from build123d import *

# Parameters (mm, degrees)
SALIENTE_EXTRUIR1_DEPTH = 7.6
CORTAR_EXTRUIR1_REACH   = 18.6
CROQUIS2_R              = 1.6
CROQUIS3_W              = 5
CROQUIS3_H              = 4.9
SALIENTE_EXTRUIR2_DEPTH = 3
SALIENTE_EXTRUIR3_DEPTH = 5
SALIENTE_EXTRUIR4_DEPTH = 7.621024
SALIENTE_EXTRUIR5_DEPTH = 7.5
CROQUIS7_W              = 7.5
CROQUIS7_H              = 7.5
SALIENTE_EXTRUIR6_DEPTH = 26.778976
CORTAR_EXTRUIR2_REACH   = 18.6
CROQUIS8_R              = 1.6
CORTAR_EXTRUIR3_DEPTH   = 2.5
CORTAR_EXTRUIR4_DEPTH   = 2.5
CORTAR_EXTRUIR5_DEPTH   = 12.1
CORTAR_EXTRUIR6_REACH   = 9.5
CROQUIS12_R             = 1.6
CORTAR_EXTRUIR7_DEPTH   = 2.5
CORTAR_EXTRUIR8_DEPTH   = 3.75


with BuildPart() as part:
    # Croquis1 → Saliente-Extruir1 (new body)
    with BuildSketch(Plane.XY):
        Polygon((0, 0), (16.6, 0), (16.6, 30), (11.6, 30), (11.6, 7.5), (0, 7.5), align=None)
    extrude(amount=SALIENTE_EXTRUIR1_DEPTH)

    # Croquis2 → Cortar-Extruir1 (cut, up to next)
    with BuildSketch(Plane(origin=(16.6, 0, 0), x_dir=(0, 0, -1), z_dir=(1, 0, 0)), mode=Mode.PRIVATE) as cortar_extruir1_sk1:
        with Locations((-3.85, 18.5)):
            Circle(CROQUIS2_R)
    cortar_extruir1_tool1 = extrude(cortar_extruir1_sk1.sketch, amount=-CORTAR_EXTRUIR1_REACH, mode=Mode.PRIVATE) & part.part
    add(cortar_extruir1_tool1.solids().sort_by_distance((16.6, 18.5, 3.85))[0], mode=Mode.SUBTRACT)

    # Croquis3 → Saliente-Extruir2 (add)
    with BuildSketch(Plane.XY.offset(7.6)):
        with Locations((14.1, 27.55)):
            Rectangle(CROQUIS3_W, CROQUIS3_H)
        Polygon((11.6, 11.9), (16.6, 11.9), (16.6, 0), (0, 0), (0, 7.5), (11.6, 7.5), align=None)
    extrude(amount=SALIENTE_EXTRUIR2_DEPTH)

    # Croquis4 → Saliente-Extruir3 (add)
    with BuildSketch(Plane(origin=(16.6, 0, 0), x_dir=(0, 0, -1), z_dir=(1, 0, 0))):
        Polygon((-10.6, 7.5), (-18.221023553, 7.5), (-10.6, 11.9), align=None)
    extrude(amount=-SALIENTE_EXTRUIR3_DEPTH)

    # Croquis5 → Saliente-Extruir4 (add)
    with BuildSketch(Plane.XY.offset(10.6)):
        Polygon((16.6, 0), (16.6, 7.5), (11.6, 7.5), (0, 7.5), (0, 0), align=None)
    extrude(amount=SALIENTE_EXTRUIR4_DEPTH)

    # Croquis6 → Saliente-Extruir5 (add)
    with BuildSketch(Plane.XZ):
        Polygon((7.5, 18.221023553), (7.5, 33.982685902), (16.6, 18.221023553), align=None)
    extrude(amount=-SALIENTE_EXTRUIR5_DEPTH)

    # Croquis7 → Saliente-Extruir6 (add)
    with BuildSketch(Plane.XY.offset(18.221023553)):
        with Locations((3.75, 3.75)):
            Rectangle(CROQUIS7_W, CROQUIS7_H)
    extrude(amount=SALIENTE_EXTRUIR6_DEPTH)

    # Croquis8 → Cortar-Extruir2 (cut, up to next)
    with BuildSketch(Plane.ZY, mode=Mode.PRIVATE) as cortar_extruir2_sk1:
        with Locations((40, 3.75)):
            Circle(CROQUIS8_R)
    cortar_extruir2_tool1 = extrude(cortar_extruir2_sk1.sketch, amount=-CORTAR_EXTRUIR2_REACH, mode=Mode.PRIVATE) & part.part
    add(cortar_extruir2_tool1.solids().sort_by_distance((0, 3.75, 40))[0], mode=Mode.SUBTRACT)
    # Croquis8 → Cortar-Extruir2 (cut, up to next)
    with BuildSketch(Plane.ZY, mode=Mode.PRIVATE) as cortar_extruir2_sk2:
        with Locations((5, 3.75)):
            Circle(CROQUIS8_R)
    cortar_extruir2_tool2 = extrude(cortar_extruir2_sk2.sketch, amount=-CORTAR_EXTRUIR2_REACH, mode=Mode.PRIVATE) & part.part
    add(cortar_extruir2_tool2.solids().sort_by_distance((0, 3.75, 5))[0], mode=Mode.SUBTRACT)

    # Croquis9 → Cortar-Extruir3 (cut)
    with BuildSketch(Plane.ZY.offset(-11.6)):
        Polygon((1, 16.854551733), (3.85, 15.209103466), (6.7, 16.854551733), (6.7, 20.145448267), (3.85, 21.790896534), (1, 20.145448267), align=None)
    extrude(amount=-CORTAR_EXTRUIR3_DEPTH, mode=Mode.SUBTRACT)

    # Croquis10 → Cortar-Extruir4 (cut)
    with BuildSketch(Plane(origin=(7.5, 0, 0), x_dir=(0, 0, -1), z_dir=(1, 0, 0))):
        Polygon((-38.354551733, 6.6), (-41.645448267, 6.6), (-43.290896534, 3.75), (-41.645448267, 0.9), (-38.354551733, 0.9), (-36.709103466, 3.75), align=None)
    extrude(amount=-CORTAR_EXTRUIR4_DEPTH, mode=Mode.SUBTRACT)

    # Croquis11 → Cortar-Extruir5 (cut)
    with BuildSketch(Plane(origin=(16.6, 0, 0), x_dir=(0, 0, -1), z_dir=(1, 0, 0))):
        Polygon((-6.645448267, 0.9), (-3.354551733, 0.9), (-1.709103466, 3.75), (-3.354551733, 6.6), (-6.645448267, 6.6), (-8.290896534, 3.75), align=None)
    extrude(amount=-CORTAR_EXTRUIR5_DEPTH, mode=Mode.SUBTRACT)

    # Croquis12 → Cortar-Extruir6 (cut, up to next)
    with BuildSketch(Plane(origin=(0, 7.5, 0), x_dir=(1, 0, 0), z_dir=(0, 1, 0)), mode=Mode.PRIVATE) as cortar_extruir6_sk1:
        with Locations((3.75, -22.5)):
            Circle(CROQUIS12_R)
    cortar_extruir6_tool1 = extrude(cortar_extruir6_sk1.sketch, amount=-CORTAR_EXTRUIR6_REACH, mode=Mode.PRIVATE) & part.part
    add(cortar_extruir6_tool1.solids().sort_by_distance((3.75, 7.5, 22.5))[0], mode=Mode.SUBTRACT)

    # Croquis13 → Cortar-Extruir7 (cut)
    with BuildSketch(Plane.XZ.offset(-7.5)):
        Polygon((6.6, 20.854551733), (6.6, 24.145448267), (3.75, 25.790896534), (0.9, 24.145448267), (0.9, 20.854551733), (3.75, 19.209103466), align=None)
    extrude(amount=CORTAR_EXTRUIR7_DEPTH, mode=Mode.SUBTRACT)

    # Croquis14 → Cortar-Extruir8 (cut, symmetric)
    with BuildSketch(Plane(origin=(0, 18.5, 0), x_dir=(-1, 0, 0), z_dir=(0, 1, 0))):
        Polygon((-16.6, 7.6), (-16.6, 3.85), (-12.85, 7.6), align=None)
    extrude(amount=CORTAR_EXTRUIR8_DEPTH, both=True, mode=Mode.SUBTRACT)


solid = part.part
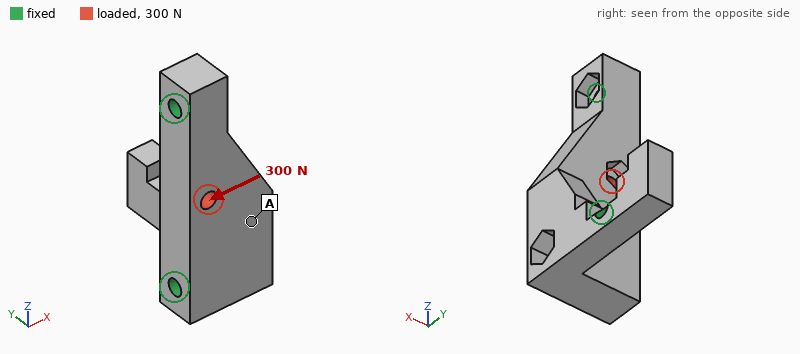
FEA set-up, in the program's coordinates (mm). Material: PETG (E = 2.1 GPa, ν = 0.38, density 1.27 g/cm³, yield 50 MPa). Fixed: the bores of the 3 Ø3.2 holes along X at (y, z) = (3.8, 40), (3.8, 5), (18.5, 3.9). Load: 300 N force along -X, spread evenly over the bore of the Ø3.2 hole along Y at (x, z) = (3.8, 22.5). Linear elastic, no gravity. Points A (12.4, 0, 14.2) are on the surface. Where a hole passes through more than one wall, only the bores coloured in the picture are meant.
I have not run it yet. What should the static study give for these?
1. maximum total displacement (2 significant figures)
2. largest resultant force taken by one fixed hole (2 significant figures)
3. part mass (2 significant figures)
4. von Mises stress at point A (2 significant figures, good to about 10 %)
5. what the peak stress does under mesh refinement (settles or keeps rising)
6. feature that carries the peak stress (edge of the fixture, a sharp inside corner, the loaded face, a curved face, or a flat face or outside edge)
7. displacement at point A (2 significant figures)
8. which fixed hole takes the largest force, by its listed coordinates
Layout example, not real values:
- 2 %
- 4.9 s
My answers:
- 0.13 mm
- 200 N
- 5.9 g
- 3.4 MPa
- keeps rising
- edge of the fixture
- 0.060 mm
- (3.8, 5)
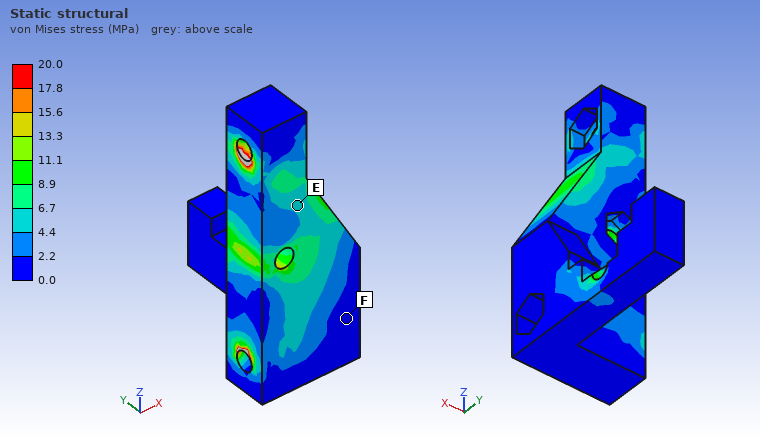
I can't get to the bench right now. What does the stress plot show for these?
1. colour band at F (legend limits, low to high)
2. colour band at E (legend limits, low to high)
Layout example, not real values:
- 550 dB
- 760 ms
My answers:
- 0.0 to 2.2 MPa
- 4.4 to 6.7 MPa
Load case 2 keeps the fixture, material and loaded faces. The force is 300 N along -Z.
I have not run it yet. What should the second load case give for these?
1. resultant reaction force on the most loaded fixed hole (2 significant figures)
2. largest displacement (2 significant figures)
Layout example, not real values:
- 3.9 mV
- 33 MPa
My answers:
- 150 N
- 32 µm
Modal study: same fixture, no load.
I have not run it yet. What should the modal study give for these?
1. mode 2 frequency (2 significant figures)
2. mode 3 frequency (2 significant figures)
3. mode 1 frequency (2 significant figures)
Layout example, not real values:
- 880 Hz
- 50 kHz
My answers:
- 4600 Hz
- 4700 Hz
- 3400 Hz
